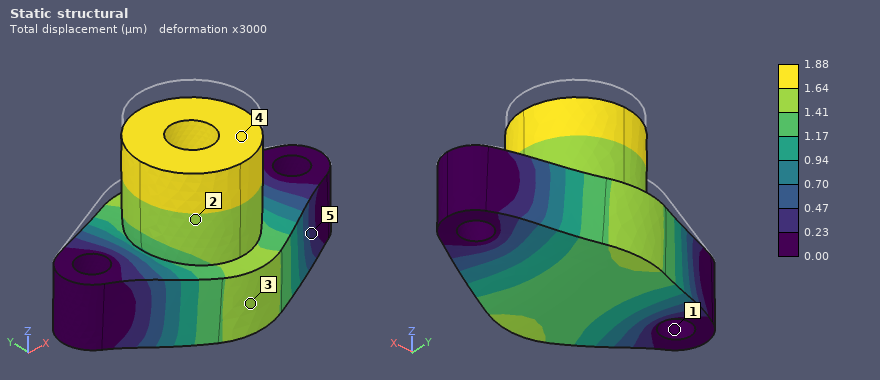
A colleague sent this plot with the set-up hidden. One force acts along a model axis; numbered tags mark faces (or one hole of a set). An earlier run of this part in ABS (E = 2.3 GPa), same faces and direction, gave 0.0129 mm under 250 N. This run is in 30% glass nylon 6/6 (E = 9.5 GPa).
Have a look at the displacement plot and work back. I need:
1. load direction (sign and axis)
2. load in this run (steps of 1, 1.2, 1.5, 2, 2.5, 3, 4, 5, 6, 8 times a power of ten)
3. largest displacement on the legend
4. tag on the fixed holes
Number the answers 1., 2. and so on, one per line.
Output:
1. -Z
2. 150 N
3. 1.88 µm
4. 1
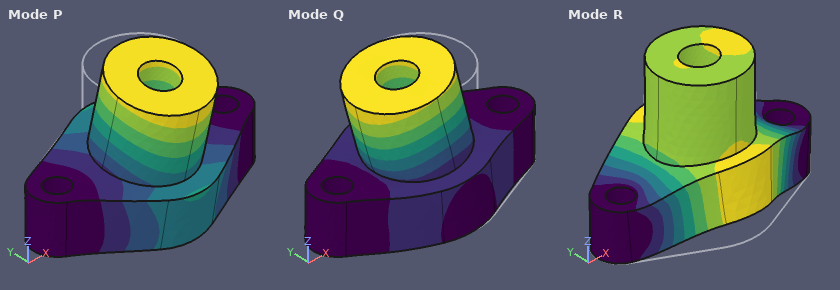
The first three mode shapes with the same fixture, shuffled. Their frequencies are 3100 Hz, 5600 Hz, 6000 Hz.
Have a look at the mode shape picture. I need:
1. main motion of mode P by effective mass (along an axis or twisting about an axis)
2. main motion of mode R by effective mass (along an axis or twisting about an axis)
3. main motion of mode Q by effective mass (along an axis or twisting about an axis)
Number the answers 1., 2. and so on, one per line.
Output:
1. along Y
2. along Z
3. along X
